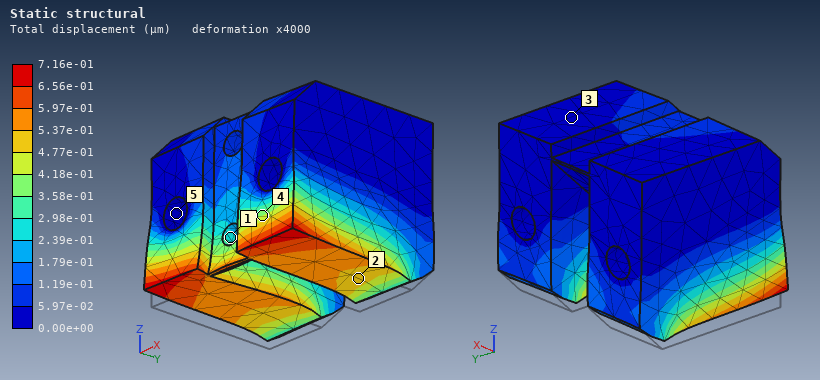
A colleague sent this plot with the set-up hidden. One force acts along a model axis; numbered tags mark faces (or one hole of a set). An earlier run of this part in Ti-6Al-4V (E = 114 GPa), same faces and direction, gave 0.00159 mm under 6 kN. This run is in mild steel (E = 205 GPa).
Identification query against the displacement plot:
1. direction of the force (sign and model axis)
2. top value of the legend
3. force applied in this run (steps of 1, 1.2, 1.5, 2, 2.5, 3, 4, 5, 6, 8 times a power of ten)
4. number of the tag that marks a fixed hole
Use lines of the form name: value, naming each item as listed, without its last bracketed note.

direction of the force: +Z
top value of the legend: 7.16e-01 µm
force applied in this run: 5 kN
number of the tag that marks a fixed hole: 5
